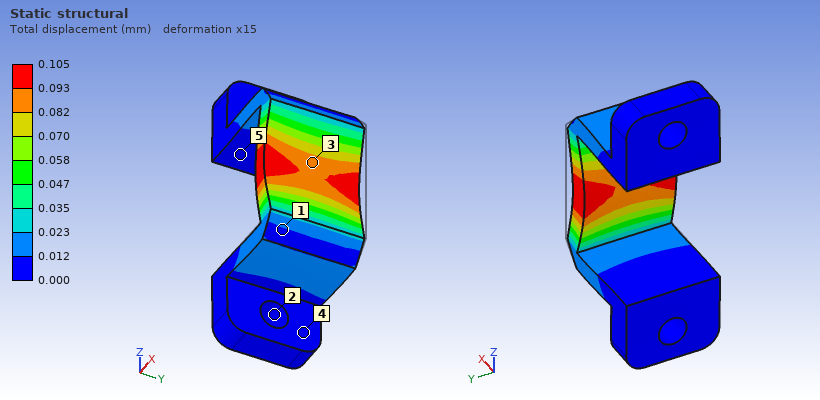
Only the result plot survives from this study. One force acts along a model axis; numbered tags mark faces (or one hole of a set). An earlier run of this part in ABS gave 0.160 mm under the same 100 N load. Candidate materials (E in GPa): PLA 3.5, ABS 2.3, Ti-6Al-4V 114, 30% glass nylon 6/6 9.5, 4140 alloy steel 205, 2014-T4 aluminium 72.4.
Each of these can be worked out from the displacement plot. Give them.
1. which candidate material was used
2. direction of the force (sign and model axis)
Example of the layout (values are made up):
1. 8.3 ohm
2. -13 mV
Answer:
1. PLA
2. -X
